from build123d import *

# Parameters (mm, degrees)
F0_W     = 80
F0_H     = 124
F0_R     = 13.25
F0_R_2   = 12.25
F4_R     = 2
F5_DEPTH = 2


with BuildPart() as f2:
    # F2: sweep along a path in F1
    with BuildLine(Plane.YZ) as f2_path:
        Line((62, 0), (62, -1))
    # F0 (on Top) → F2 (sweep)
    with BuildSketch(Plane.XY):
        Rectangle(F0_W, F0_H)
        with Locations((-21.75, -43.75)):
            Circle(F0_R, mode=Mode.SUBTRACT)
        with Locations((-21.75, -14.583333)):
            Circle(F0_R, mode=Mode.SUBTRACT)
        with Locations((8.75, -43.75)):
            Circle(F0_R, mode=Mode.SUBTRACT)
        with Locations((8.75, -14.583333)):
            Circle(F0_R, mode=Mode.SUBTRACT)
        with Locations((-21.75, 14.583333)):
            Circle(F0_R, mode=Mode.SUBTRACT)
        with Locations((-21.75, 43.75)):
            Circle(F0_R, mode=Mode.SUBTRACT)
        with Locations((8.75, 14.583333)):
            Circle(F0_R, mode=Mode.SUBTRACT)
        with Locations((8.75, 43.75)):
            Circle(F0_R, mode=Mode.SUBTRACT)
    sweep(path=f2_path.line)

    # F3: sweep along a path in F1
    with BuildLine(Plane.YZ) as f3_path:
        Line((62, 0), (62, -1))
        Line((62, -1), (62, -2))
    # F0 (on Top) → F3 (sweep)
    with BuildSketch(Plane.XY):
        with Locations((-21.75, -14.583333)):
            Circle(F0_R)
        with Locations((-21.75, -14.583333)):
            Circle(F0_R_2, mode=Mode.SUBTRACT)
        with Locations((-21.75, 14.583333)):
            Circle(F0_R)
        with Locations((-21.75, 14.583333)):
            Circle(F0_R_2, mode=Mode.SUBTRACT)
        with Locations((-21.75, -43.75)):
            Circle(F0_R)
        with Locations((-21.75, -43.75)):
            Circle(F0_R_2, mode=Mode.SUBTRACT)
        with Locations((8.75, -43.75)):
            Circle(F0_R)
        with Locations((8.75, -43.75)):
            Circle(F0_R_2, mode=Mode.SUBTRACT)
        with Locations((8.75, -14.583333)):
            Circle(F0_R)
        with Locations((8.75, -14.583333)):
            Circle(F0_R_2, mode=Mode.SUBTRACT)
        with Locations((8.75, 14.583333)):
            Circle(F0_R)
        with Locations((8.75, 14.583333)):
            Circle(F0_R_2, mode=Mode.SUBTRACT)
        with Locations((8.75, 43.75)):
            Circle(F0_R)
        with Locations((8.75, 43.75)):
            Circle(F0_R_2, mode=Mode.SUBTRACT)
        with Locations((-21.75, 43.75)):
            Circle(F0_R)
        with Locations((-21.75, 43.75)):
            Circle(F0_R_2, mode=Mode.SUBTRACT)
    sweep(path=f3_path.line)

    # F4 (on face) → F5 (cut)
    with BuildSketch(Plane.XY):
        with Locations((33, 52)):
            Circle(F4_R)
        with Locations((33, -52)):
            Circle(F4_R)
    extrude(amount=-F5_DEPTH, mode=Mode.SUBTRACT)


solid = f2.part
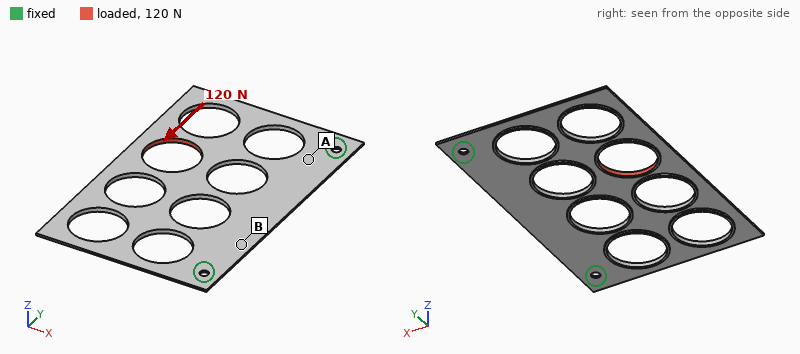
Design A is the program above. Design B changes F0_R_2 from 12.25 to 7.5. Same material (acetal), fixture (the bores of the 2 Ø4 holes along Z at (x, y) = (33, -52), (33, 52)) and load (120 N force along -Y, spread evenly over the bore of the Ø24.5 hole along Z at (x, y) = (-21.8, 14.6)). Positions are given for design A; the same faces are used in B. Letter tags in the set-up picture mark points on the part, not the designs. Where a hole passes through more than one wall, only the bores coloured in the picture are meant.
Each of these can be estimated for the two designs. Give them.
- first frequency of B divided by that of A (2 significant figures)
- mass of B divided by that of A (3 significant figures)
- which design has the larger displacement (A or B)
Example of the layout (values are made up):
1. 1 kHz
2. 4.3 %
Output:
1. 0.90
2. 1.70
3. A
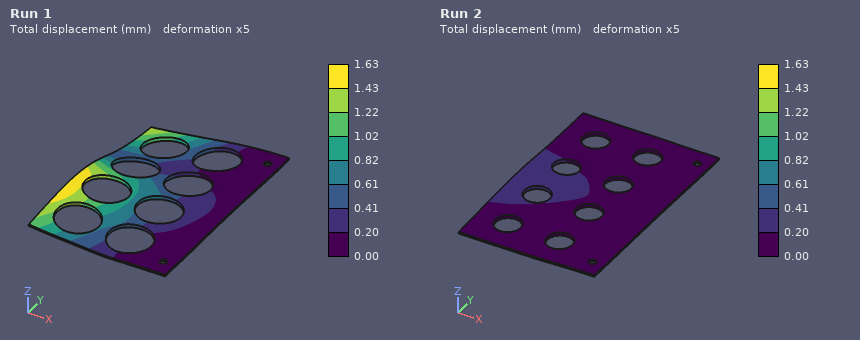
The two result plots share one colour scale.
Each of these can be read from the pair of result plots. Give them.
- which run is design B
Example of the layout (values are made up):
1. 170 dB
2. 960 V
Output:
1. Run 2
